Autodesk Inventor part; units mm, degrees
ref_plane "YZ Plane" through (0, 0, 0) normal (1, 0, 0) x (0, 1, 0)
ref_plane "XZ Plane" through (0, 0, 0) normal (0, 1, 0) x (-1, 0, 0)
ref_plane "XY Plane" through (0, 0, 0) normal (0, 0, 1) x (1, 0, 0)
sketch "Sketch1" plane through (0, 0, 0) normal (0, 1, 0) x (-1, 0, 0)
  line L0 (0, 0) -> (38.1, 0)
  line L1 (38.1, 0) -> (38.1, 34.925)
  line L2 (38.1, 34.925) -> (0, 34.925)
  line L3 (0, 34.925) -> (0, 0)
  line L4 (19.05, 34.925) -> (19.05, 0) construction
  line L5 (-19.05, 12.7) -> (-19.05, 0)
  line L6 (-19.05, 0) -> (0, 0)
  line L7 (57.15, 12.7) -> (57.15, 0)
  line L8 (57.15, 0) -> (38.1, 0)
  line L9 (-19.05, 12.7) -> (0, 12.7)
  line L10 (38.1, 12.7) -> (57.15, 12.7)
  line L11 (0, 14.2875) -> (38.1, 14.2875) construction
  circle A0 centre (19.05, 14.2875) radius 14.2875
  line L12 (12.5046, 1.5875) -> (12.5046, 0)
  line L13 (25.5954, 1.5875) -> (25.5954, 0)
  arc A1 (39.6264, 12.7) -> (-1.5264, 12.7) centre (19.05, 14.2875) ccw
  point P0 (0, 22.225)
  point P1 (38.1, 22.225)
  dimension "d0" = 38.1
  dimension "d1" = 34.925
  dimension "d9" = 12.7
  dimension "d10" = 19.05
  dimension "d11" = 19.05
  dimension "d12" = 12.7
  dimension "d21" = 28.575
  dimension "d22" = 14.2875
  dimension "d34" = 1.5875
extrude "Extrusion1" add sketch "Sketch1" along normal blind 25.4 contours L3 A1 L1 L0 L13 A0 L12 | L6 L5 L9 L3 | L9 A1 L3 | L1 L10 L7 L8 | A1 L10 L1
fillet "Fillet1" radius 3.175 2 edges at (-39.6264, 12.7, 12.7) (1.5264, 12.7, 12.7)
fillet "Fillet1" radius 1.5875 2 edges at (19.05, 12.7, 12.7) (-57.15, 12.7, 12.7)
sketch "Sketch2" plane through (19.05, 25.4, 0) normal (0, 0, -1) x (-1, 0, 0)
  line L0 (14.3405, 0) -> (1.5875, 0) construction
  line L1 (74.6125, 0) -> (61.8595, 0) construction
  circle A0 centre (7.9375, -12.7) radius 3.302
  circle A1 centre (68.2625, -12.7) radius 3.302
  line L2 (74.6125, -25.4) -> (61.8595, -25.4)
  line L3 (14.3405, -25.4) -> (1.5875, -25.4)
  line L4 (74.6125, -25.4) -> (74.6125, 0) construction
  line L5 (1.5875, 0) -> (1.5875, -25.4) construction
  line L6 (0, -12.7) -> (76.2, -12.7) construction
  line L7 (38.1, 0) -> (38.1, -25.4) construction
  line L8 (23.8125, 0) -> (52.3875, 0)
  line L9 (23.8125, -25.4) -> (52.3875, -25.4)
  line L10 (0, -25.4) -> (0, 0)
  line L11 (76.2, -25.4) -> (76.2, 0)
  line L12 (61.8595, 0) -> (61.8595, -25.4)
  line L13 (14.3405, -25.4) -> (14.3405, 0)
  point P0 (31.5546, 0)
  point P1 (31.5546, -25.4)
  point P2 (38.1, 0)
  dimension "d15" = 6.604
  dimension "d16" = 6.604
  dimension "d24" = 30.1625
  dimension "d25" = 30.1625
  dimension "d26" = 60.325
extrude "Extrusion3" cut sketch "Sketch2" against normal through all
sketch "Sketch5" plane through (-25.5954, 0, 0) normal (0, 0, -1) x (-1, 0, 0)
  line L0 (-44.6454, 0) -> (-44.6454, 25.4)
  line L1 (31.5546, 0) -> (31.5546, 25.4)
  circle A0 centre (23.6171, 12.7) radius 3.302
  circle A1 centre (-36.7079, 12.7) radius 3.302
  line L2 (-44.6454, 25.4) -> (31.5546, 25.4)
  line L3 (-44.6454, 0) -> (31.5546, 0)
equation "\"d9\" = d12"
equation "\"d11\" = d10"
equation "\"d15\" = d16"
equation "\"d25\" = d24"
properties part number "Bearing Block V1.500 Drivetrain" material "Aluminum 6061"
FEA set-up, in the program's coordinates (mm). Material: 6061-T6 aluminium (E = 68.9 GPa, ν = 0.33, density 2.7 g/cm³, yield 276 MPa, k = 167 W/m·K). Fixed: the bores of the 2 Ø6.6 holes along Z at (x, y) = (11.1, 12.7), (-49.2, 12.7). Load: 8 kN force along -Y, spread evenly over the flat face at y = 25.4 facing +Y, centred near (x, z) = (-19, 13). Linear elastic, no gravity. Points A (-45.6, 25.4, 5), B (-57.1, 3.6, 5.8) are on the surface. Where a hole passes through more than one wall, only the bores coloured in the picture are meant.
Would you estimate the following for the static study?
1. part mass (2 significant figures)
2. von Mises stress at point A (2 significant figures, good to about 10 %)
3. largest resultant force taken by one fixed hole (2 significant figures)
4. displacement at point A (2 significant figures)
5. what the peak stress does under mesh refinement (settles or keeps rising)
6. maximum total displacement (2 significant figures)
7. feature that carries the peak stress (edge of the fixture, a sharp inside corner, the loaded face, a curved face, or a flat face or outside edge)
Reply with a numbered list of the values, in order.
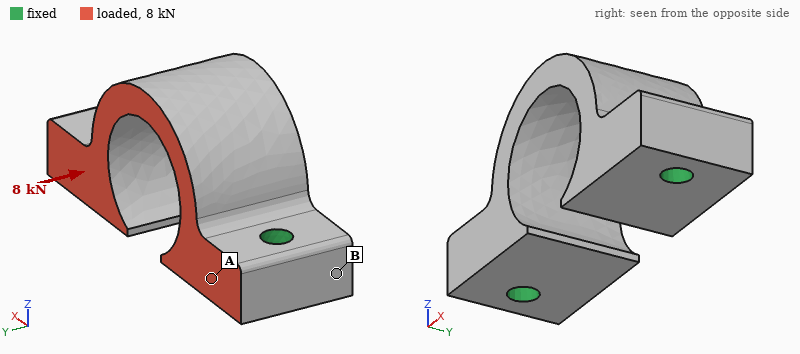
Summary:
1. 70 g
2. 30 MPa
3. 4.0 kN
4. 12 µm
5. keeps rising
6. 61 µm
7. edge of the fixture
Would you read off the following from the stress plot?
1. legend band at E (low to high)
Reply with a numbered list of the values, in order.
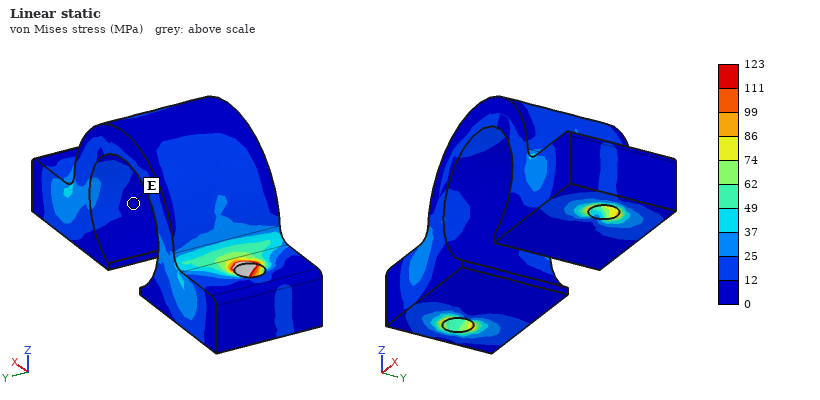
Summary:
1. 0 to 12 MPa
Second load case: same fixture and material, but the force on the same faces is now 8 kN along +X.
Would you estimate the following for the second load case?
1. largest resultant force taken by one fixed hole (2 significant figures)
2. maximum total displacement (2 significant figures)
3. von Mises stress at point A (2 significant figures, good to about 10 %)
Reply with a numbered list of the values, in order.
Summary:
1. 4.1 kN
2. 41 µm
3. 16 MPa
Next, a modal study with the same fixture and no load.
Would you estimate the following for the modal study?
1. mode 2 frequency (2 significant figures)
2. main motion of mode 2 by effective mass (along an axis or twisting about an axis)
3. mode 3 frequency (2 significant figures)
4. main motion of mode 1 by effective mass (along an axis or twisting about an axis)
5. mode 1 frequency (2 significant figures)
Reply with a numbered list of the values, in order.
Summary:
1. 12 kHz
2. along X
3. 16 kHz
4. along Y
5. 8300 Hz
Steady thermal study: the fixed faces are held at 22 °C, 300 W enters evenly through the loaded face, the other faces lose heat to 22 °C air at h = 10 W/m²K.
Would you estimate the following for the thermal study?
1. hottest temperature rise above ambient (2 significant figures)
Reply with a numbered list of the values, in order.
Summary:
1. 70 K
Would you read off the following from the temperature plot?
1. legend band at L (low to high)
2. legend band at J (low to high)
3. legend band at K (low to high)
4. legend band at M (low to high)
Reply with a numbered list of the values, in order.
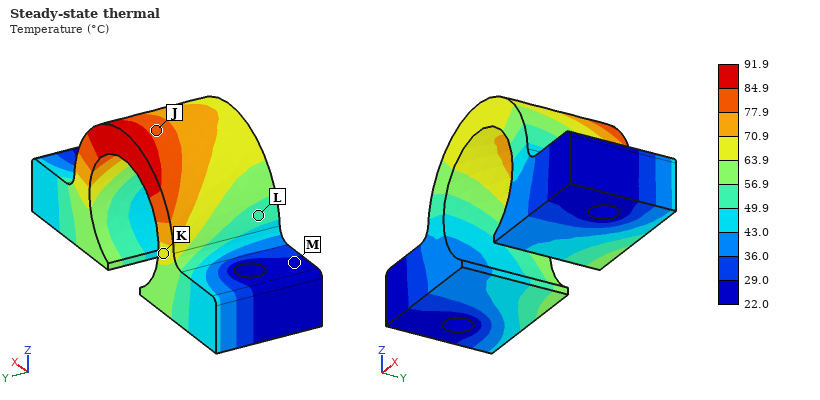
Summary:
1. 49.9 to 56.9 °C
2. 77.9 to 84.9 °C
3. 63.9 to 70.9 °C
4. 22.0 to 29.0 °C
